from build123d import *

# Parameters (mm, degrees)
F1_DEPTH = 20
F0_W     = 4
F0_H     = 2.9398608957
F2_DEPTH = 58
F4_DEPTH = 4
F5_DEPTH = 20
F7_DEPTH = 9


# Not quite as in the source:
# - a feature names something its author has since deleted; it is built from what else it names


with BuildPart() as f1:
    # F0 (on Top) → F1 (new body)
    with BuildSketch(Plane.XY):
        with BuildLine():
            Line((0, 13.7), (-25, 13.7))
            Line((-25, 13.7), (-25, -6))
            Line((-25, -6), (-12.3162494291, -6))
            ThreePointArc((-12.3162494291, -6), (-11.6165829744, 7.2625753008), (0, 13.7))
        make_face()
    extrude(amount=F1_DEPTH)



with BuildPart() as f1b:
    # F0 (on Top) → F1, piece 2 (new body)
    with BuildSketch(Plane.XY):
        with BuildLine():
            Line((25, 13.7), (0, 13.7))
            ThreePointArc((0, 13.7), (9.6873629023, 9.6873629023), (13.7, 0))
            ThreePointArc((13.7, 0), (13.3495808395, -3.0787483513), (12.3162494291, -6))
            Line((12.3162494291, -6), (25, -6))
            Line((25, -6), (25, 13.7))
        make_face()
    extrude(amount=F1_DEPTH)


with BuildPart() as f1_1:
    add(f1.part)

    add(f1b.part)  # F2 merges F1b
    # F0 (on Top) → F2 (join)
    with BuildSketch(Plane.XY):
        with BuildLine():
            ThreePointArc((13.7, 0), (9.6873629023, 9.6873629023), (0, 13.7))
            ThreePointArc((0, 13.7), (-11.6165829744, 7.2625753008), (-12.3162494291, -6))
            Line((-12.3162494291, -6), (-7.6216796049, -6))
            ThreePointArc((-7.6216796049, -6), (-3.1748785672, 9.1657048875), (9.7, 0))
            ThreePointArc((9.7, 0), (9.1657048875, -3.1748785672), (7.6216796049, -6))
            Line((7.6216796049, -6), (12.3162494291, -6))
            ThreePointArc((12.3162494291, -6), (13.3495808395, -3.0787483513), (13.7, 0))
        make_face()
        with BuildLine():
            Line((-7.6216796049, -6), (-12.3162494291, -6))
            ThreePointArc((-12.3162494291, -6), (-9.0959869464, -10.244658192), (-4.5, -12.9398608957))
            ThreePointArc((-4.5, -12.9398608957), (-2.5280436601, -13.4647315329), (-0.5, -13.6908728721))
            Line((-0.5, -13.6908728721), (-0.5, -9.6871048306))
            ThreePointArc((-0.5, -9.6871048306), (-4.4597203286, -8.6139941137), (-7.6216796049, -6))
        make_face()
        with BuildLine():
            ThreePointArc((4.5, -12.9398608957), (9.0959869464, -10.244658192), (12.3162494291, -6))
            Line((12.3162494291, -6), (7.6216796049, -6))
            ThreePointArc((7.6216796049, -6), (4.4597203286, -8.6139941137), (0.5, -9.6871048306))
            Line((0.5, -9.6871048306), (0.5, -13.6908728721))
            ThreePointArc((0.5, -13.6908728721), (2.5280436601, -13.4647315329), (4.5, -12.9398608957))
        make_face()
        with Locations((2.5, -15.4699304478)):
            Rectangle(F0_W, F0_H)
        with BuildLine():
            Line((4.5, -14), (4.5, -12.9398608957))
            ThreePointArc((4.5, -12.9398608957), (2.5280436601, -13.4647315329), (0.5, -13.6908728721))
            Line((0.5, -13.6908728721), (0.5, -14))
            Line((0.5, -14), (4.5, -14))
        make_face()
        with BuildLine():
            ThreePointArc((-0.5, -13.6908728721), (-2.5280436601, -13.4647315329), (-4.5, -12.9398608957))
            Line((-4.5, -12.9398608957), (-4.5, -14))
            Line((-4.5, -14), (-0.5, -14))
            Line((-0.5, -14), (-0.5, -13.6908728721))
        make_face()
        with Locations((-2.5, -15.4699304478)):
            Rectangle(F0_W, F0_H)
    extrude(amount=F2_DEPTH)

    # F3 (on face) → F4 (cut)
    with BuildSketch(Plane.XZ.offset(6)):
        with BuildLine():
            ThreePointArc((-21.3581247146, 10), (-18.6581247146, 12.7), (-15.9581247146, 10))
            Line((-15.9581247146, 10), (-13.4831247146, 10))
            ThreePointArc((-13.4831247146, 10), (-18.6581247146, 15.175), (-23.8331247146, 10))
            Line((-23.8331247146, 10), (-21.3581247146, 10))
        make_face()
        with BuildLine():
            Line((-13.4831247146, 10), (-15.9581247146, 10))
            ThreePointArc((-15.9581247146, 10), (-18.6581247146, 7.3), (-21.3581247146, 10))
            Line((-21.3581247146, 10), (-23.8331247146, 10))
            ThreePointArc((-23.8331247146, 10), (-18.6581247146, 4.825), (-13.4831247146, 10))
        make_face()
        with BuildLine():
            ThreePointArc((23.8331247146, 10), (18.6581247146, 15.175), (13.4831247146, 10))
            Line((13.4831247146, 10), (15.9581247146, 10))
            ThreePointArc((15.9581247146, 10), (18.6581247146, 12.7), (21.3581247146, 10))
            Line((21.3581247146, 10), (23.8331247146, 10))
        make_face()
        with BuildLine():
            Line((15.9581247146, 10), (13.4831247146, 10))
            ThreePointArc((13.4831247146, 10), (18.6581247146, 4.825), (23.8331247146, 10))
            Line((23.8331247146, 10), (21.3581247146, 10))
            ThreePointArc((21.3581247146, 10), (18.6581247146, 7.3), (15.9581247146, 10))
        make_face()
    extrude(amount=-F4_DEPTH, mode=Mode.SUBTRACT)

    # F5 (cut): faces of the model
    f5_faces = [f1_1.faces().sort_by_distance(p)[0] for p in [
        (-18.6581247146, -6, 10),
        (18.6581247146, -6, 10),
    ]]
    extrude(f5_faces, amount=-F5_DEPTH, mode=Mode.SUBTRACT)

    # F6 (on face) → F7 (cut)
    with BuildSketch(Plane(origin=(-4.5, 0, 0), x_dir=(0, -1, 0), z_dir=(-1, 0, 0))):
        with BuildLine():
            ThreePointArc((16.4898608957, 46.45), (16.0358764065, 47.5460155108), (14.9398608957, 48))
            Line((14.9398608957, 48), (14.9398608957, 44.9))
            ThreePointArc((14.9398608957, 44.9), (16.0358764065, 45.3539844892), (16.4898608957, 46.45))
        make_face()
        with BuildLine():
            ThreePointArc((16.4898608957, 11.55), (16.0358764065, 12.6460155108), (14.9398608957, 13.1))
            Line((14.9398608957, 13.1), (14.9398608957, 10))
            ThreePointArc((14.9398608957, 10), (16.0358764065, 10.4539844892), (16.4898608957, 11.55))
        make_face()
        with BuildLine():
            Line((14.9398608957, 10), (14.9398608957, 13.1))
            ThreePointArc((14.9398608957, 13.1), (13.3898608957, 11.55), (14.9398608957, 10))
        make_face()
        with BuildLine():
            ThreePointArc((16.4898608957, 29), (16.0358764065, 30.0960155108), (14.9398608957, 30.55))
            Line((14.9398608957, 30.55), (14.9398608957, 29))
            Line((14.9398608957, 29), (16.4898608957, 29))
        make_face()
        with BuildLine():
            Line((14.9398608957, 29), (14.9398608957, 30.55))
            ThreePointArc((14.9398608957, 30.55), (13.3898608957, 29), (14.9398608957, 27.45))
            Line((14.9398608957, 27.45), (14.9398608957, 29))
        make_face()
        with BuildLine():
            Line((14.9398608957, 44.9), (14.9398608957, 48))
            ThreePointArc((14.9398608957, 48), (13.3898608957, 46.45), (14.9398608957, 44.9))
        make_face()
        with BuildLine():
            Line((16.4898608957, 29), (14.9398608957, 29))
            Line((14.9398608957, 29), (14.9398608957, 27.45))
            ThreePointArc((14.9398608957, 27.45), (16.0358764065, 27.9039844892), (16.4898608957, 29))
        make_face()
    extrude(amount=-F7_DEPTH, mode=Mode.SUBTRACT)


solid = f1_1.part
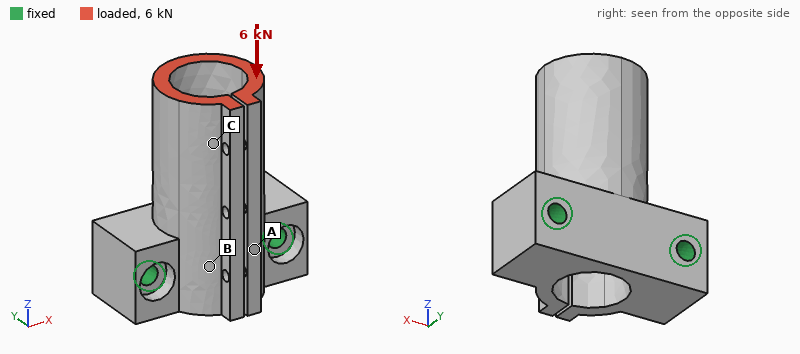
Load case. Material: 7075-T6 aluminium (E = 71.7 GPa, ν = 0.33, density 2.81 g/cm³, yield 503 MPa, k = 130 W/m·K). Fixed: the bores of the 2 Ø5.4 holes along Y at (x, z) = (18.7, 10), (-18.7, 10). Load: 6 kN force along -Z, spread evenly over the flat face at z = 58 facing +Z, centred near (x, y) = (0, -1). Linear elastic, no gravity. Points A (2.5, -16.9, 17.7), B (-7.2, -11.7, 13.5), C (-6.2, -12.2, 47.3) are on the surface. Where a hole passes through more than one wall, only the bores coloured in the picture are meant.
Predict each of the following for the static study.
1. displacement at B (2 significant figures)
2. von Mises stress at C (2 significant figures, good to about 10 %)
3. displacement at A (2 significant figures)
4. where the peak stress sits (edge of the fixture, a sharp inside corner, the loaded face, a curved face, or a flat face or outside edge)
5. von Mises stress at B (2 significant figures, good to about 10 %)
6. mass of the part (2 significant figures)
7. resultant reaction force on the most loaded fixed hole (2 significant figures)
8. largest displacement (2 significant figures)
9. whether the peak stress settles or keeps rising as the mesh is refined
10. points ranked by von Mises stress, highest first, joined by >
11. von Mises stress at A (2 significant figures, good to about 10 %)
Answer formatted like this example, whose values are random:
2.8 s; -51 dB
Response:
20 µm; 24 MPa; 30 µm; edge of the fixture; 16 MPa; 77 g; 3.0 kN; 62 µm; keeps rising; C > B > A; 6.8 MPa
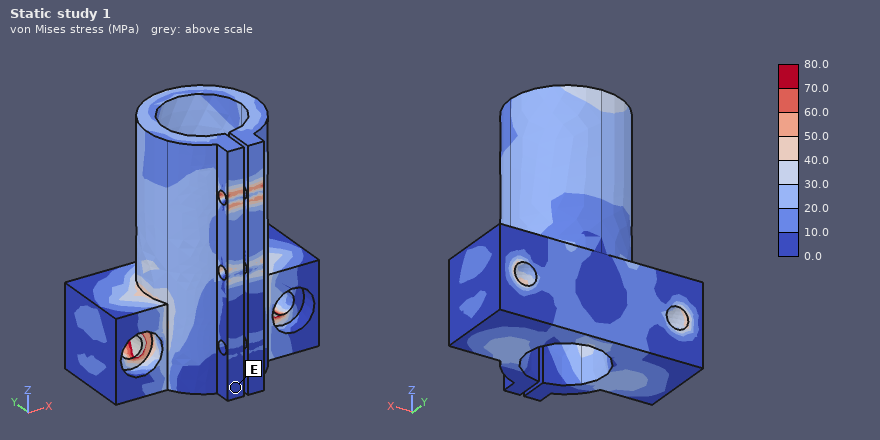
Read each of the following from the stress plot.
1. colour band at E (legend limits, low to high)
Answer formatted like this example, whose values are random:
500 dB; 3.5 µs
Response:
0.0 to 10.0 MPa
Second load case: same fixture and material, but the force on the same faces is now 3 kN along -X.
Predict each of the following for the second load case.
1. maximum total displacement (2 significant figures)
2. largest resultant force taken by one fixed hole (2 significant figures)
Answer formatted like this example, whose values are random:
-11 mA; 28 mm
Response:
0.42 mm; 3.5 kN
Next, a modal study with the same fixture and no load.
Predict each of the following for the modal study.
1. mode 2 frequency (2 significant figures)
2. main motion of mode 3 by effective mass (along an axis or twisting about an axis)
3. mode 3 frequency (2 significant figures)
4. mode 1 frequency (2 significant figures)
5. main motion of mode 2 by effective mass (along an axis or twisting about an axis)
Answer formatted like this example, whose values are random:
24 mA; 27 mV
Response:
4400 Hz; along Y; 5800 Hz; 4100 Hz; along X
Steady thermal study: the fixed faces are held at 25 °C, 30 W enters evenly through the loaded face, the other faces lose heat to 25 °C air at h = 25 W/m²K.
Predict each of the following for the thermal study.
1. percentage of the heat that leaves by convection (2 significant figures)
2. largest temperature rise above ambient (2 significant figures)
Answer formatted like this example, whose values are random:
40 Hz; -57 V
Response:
12 %; 34 K
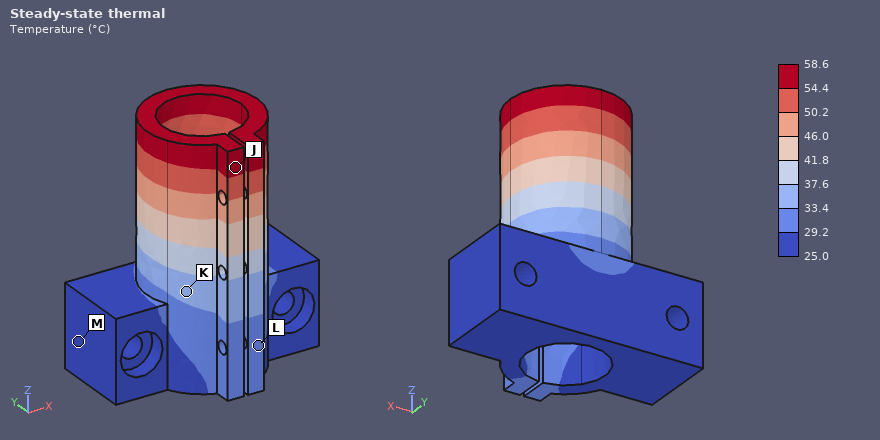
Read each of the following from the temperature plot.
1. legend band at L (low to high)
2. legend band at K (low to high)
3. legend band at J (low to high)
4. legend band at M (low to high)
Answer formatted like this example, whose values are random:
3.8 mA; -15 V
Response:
29.2 to 33.4 °C; 33.4 to 37.6 °C; 54.4 to 58.6 °C; 25.0 to 29.2 °C
